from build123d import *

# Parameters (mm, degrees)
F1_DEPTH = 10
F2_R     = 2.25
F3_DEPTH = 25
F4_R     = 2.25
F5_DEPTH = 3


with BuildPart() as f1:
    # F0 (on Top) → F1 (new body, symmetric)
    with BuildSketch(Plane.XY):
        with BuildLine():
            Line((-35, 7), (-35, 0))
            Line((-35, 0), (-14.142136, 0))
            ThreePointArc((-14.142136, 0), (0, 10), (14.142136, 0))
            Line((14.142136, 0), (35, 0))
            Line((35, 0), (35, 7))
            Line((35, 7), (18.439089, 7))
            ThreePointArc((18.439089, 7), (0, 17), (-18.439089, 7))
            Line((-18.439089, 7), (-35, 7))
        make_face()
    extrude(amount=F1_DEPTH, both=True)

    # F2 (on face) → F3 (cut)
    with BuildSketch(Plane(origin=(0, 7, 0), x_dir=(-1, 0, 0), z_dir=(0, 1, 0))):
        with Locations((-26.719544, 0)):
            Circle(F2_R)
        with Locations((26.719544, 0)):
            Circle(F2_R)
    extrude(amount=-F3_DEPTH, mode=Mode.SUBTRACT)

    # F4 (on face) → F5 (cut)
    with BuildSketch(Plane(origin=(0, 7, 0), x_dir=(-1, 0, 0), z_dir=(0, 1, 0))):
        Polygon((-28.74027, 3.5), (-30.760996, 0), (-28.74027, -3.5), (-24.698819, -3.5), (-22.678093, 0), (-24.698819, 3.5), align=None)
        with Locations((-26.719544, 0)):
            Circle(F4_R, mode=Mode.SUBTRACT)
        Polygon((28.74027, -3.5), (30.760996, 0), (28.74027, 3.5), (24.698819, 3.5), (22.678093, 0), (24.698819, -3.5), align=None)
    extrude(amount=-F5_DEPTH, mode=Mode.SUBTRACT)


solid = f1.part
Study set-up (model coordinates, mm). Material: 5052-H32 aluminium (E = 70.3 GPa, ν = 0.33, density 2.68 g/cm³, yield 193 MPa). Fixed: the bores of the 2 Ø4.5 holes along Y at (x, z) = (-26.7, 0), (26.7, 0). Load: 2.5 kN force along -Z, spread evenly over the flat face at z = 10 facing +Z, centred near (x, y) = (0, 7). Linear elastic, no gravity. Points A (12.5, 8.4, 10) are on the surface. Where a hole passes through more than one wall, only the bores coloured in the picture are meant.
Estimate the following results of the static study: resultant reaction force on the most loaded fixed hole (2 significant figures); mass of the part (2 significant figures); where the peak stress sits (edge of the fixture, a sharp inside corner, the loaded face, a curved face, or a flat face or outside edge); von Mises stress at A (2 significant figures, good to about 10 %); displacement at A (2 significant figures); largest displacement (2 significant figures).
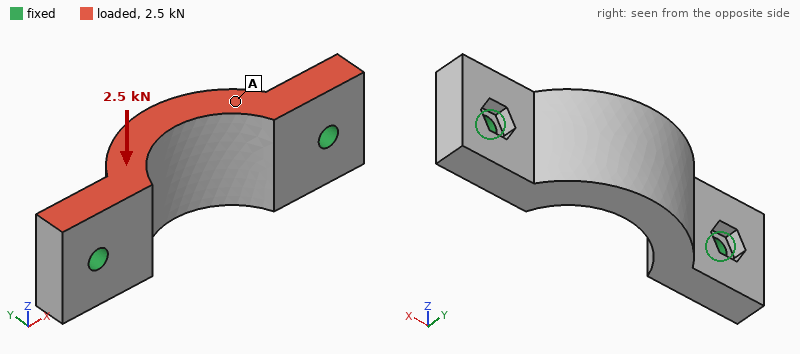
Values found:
1.3 kN
28 g
edge of the fixture
19 MPa
35 µm
58 µm
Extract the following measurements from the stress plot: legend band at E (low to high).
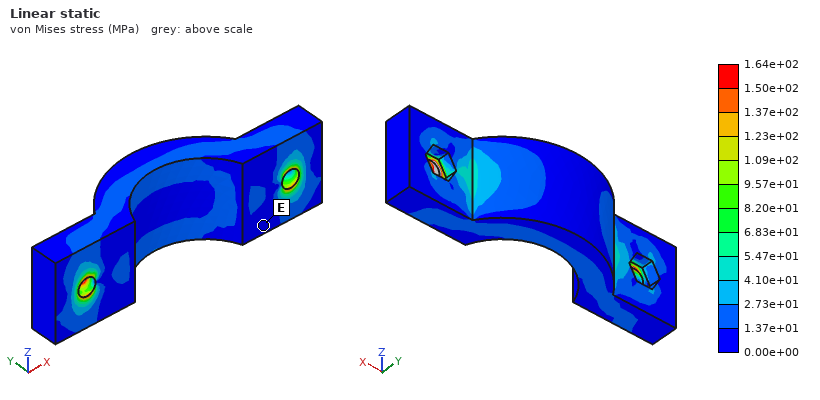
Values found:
0.00e+00 to 1.37e+01 MPa
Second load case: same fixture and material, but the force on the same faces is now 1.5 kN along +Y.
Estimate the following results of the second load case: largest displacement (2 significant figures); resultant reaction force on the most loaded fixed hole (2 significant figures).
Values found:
50 µm
900 N
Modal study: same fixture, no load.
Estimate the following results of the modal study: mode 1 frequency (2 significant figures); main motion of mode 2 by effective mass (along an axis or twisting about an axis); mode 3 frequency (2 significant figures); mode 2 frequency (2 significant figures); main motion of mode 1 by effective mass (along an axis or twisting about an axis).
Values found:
7300 Hz
along Y
19 kHz
14 kHz
along Z
